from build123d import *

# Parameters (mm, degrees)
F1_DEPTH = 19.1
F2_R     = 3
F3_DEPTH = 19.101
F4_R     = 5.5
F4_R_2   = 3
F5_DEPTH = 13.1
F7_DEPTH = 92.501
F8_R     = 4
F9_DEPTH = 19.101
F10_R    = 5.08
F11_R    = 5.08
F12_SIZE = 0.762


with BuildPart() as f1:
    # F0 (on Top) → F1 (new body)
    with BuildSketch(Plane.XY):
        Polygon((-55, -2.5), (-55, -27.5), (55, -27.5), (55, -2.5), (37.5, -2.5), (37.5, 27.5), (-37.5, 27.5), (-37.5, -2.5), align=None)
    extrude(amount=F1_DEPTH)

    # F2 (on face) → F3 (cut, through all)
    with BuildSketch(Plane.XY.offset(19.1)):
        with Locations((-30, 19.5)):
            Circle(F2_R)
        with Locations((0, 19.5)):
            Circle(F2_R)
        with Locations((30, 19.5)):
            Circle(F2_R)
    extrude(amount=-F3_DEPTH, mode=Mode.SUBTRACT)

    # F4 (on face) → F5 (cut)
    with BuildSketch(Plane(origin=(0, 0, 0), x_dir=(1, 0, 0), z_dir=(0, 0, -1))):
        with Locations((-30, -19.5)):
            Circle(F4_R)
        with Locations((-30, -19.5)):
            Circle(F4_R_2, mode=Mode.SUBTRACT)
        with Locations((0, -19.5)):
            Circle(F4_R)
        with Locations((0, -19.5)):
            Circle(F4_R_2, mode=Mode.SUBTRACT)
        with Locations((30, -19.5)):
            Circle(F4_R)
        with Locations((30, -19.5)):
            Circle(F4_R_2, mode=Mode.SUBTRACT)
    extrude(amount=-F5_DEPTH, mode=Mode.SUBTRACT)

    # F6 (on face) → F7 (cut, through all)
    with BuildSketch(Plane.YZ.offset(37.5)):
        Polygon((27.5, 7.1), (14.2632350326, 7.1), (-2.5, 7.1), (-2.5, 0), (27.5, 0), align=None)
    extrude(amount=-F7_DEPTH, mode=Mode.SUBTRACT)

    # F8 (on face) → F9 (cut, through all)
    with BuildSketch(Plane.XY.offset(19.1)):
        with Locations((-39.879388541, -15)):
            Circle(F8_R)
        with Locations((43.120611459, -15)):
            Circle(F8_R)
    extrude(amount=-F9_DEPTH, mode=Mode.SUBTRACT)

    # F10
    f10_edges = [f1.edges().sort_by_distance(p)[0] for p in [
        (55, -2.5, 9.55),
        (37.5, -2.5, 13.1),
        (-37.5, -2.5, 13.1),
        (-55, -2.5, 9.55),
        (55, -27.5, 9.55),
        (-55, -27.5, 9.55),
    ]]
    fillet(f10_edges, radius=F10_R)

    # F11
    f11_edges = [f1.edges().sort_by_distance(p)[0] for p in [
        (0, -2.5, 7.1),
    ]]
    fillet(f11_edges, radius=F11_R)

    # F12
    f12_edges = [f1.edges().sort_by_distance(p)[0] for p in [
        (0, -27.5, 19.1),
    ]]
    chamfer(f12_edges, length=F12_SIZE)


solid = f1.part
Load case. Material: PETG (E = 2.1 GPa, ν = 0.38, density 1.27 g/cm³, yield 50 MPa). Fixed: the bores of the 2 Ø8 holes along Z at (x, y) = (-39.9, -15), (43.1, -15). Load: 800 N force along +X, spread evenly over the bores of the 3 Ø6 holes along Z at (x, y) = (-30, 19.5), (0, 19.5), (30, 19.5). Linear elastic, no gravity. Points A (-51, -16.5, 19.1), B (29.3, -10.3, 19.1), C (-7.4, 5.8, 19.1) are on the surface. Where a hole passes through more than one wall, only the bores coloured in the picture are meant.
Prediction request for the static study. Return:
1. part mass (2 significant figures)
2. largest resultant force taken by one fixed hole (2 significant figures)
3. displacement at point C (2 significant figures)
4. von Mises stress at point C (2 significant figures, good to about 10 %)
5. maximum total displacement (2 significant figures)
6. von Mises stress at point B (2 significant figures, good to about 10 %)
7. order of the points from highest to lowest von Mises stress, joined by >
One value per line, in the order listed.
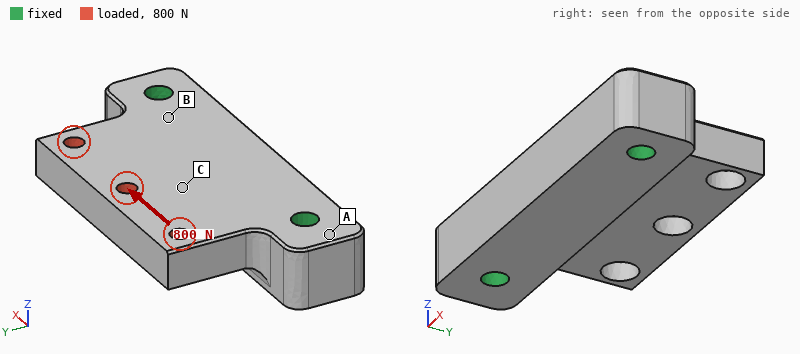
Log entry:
96 g
530 N
27 µm
1.8 MPa
78 µm
0.99 MPa
C > B > A
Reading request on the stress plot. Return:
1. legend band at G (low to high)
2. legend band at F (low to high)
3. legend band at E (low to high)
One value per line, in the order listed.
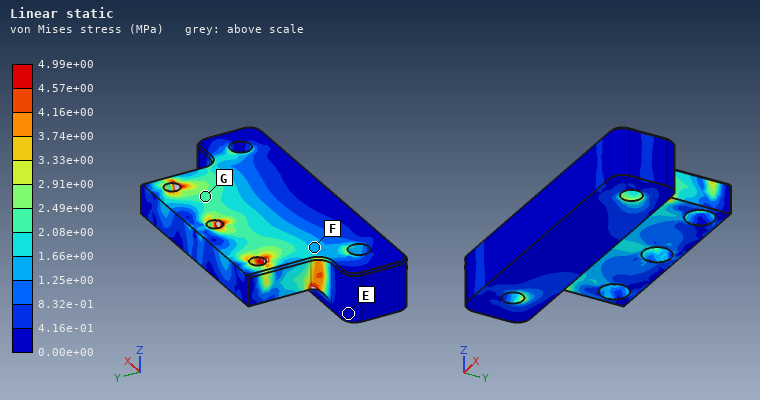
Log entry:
2.08e+00 to 2.49e+00 MPa
1.25e+00 to 1.66e+00 MPa
0.00e+00 to 4.16e-01 MPa
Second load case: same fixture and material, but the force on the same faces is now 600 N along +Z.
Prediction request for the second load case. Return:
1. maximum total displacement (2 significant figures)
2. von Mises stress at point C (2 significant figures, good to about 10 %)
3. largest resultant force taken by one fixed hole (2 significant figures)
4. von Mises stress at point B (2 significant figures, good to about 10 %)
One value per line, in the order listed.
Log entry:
0.49 mm
3.6 MPa
310 N
4.8 MPa
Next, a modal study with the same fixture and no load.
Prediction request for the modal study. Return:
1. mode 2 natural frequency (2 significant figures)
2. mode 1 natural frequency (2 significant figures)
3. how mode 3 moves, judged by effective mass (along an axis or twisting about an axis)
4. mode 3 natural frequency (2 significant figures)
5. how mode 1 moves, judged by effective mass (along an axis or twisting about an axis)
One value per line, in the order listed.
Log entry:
2600 Hz
1400 Hz
along Z
2900 Hz
along Z
